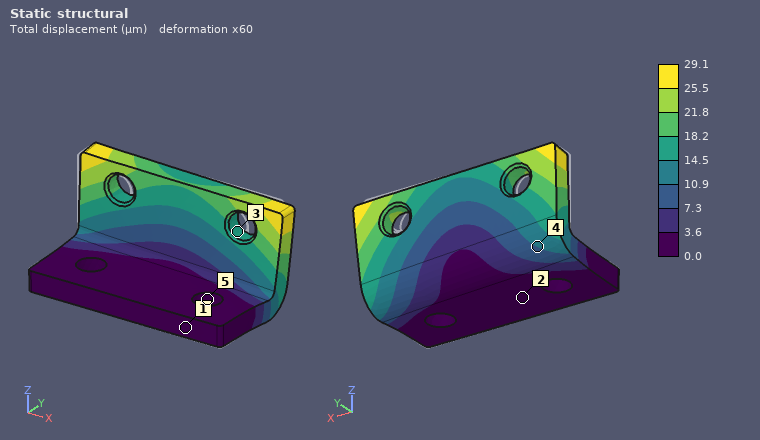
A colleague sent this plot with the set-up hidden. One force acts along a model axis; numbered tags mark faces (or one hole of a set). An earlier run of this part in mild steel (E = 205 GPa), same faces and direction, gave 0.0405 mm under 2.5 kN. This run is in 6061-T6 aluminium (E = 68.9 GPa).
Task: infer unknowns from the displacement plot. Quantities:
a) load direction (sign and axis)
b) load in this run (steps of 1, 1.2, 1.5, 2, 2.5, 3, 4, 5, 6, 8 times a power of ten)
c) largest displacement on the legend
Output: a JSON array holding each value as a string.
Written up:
["+X", "600 N", "29.1 µm"]
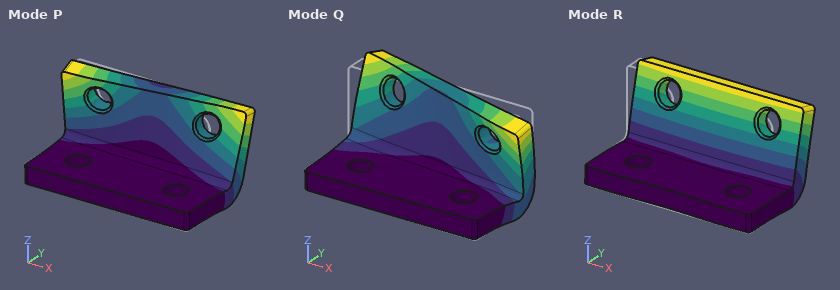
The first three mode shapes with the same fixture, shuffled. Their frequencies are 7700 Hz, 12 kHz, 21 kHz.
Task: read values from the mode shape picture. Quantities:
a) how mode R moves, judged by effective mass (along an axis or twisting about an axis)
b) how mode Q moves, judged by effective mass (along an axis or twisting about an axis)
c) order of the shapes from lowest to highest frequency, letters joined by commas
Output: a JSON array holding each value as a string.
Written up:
["along Y", "along X", "R, P, Q"]
